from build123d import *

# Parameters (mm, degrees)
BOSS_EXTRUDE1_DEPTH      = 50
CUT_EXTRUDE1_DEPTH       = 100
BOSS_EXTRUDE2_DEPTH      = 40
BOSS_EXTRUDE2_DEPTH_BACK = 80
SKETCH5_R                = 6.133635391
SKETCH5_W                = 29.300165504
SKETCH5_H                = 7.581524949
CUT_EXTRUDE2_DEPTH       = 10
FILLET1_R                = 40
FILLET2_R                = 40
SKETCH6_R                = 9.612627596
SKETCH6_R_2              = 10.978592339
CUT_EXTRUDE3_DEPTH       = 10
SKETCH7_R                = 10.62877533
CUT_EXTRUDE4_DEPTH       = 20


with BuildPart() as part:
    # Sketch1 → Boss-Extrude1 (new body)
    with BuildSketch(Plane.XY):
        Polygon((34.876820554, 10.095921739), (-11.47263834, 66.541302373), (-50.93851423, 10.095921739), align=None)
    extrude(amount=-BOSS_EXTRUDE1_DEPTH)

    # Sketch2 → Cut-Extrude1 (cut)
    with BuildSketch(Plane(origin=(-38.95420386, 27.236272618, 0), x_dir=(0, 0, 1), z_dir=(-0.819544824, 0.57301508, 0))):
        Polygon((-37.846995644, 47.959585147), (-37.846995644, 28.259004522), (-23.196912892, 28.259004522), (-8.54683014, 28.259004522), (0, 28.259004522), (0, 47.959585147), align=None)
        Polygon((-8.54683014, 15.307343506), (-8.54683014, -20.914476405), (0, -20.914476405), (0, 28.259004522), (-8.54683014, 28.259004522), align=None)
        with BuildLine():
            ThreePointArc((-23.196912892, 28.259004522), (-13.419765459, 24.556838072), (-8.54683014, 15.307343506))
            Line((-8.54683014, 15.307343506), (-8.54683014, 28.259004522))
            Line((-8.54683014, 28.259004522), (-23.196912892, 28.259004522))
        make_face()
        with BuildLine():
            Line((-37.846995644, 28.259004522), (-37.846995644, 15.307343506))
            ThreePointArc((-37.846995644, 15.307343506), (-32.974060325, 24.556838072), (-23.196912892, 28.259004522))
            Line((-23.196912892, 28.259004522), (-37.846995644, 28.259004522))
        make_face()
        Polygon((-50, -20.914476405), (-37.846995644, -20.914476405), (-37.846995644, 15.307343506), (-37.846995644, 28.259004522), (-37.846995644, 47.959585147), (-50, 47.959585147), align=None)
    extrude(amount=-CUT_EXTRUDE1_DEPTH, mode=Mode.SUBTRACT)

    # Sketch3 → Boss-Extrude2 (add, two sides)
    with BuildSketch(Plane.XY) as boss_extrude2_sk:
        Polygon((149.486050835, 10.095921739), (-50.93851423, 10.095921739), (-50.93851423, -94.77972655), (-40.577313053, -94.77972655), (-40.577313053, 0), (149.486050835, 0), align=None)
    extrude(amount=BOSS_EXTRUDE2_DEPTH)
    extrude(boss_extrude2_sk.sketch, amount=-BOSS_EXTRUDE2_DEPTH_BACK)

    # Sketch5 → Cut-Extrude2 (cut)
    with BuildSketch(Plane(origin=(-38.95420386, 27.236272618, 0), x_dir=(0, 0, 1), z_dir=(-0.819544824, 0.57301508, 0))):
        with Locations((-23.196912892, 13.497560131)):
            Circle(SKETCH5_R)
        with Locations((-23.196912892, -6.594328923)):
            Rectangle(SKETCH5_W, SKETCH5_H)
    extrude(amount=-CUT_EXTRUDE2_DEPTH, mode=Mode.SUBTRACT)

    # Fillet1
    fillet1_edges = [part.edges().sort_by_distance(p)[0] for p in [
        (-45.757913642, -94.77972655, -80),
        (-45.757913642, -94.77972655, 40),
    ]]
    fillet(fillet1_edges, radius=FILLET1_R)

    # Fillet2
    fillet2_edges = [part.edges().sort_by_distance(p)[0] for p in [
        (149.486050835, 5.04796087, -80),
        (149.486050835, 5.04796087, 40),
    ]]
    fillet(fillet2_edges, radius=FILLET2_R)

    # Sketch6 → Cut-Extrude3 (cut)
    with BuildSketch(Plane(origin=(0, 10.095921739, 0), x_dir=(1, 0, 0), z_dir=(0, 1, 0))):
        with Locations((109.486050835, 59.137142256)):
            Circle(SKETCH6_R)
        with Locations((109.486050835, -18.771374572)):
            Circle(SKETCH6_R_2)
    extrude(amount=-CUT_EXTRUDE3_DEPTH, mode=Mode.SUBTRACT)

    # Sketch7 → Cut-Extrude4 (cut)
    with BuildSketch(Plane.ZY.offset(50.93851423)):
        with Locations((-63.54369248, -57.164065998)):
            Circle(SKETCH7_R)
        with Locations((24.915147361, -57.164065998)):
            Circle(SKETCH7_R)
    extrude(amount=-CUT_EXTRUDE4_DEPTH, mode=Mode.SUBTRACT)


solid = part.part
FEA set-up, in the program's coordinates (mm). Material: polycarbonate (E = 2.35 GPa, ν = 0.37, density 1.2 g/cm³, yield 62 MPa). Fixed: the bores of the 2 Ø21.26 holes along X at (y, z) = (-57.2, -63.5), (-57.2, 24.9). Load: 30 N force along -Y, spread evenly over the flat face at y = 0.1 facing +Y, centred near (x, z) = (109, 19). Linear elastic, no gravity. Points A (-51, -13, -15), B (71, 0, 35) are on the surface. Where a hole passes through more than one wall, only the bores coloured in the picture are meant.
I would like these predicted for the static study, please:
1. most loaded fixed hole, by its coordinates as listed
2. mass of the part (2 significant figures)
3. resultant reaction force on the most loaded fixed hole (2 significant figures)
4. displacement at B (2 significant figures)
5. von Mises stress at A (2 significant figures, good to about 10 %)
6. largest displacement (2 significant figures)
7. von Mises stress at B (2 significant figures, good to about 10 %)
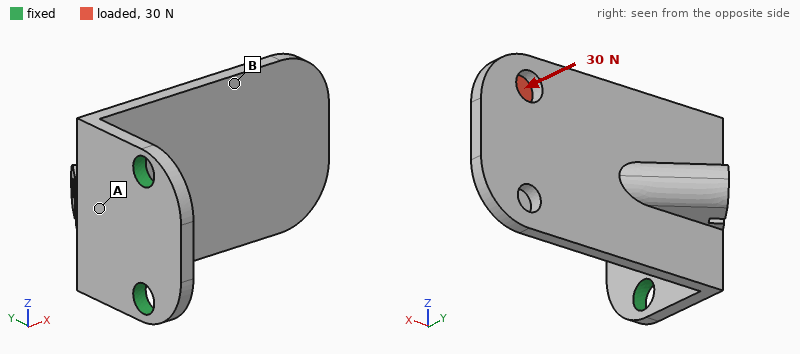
(-57.2, 24.9)
450 g
28 N
1.7 mm
2.0 MPa
3.0 mm
0.69 MPa
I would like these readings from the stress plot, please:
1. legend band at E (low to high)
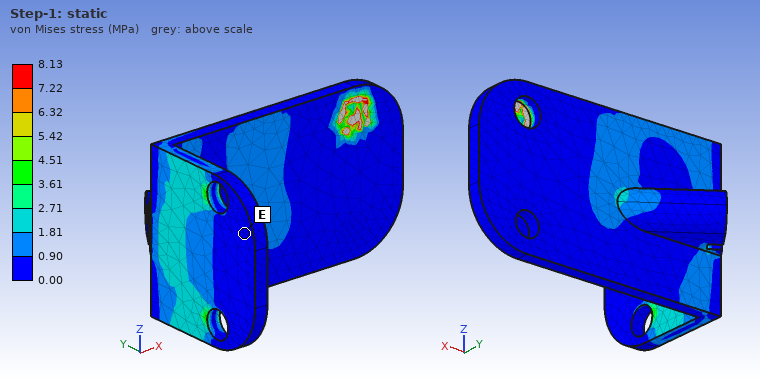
0.00 to 0.90 MPa
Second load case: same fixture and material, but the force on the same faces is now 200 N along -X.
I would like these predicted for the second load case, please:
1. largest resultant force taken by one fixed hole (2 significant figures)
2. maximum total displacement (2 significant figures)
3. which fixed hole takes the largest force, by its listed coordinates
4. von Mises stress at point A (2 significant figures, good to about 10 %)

190 N
1.7 mm
(-57.2, 24.9)
1.7 MPa
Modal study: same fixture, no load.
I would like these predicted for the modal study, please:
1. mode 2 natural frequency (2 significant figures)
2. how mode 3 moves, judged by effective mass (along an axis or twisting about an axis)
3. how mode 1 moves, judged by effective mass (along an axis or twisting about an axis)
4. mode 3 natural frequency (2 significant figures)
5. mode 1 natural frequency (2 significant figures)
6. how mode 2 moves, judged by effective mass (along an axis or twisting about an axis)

120 Hz
along X
along Y
230 Hz
52 Hz
along Z
